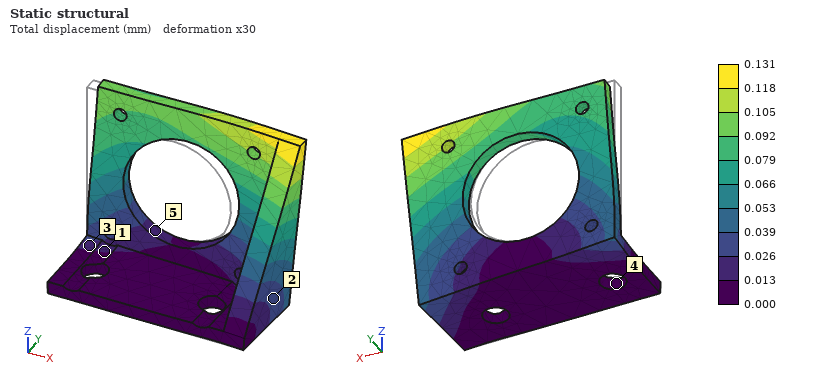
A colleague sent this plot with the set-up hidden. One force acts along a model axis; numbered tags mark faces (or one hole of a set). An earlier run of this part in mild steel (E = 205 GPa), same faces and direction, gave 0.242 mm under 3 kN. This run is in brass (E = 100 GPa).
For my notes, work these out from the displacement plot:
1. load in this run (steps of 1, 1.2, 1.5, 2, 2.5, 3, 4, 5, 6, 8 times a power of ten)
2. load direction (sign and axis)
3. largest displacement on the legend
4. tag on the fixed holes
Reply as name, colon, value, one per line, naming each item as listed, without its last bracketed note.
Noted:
load in this run: 800 N
load direction: +X
largest displacement on the legend: 0.131 mm
tag on the fixed holes: 4
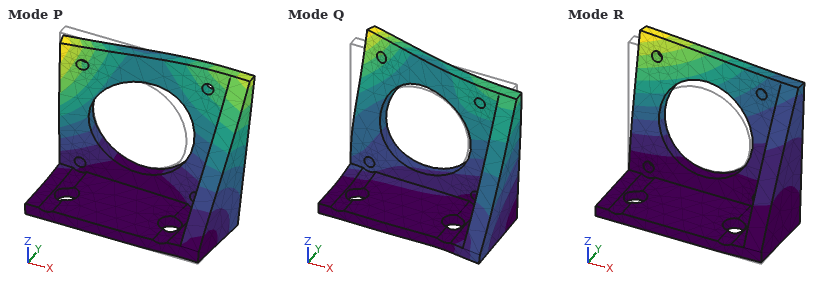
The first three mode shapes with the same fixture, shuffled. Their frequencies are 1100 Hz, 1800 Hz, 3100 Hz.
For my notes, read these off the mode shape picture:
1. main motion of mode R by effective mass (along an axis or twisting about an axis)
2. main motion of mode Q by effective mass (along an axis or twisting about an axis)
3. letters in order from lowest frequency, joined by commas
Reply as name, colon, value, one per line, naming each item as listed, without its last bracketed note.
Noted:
main motion of mode R by effective mass: along Y
main motion of mode Q by effective mass: along X
letters in order from lowest frequency, joined by commas: R, P, Q
